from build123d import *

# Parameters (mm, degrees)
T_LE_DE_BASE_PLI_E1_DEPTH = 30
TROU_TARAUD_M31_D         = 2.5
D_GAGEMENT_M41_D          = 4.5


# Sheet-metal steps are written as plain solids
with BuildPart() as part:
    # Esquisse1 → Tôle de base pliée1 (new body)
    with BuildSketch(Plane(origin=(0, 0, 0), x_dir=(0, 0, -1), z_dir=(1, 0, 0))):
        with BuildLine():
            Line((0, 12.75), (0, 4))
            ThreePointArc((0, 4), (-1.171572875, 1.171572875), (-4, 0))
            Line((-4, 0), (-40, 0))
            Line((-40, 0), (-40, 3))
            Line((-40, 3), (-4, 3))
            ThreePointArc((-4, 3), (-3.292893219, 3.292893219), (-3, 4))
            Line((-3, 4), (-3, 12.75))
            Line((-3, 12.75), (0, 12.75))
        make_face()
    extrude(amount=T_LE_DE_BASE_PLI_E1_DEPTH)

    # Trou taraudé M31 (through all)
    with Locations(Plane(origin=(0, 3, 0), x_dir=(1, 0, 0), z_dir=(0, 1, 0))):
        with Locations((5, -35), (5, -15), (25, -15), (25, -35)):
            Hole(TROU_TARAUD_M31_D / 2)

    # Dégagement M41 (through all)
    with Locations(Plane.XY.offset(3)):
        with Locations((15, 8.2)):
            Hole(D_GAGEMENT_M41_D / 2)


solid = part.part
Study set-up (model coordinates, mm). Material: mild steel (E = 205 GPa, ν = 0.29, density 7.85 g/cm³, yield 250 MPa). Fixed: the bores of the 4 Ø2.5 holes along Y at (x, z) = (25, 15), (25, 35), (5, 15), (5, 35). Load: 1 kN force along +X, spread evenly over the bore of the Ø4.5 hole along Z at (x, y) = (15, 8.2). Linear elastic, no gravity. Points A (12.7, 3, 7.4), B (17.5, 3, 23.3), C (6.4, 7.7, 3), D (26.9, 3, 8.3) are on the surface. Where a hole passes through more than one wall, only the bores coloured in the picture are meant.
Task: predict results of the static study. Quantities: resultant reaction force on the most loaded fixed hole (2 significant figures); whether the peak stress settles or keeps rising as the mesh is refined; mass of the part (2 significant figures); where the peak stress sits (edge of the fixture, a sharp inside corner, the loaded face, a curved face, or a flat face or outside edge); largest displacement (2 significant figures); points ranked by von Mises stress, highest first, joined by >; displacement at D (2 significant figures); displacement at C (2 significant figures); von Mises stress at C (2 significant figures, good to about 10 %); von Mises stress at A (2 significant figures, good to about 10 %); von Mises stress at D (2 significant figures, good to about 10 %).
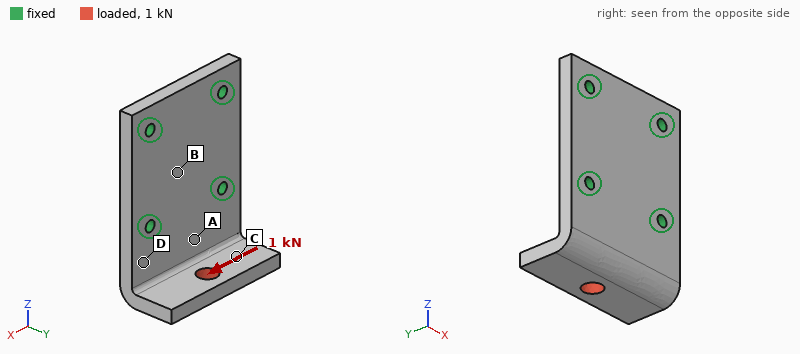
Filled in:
810 N
keeps rising
34 g
edge of the fixture
37 µm
A > D > C > B
8.6 µm
20 µm
44 MPa
87 MPa
67 MPa
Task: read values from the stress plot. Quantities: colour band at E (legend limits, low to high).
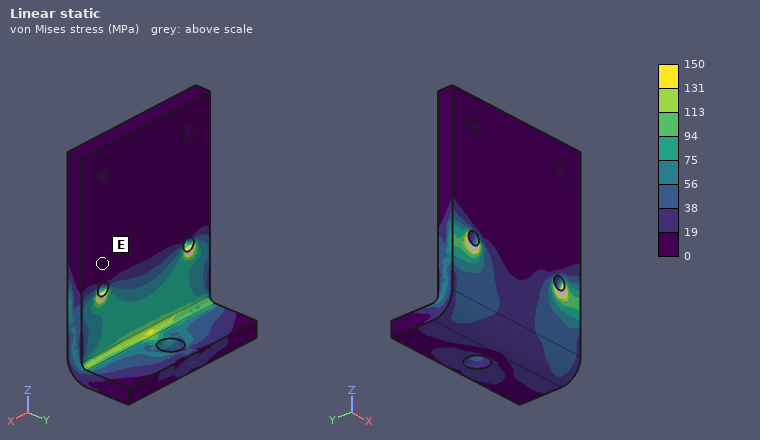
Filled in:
0 to 19 MPa
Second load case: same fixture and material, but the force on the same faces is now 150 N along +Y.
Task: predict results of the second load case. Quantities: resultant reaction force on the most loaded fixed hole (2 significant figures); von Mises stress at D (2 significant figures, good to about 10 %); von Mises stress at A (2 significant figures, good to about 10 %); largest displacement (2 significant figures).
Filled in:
88 N
22 MPa
18 MPa
17 µm
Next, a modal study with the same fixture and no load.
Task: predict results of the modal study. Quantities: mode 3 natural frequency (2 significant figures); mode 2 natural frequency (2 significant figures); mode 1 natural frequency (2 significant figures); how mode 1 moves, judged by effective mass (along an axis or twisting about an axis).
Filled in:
16 kHz
9100 Hz
5400 Hz
along Y
